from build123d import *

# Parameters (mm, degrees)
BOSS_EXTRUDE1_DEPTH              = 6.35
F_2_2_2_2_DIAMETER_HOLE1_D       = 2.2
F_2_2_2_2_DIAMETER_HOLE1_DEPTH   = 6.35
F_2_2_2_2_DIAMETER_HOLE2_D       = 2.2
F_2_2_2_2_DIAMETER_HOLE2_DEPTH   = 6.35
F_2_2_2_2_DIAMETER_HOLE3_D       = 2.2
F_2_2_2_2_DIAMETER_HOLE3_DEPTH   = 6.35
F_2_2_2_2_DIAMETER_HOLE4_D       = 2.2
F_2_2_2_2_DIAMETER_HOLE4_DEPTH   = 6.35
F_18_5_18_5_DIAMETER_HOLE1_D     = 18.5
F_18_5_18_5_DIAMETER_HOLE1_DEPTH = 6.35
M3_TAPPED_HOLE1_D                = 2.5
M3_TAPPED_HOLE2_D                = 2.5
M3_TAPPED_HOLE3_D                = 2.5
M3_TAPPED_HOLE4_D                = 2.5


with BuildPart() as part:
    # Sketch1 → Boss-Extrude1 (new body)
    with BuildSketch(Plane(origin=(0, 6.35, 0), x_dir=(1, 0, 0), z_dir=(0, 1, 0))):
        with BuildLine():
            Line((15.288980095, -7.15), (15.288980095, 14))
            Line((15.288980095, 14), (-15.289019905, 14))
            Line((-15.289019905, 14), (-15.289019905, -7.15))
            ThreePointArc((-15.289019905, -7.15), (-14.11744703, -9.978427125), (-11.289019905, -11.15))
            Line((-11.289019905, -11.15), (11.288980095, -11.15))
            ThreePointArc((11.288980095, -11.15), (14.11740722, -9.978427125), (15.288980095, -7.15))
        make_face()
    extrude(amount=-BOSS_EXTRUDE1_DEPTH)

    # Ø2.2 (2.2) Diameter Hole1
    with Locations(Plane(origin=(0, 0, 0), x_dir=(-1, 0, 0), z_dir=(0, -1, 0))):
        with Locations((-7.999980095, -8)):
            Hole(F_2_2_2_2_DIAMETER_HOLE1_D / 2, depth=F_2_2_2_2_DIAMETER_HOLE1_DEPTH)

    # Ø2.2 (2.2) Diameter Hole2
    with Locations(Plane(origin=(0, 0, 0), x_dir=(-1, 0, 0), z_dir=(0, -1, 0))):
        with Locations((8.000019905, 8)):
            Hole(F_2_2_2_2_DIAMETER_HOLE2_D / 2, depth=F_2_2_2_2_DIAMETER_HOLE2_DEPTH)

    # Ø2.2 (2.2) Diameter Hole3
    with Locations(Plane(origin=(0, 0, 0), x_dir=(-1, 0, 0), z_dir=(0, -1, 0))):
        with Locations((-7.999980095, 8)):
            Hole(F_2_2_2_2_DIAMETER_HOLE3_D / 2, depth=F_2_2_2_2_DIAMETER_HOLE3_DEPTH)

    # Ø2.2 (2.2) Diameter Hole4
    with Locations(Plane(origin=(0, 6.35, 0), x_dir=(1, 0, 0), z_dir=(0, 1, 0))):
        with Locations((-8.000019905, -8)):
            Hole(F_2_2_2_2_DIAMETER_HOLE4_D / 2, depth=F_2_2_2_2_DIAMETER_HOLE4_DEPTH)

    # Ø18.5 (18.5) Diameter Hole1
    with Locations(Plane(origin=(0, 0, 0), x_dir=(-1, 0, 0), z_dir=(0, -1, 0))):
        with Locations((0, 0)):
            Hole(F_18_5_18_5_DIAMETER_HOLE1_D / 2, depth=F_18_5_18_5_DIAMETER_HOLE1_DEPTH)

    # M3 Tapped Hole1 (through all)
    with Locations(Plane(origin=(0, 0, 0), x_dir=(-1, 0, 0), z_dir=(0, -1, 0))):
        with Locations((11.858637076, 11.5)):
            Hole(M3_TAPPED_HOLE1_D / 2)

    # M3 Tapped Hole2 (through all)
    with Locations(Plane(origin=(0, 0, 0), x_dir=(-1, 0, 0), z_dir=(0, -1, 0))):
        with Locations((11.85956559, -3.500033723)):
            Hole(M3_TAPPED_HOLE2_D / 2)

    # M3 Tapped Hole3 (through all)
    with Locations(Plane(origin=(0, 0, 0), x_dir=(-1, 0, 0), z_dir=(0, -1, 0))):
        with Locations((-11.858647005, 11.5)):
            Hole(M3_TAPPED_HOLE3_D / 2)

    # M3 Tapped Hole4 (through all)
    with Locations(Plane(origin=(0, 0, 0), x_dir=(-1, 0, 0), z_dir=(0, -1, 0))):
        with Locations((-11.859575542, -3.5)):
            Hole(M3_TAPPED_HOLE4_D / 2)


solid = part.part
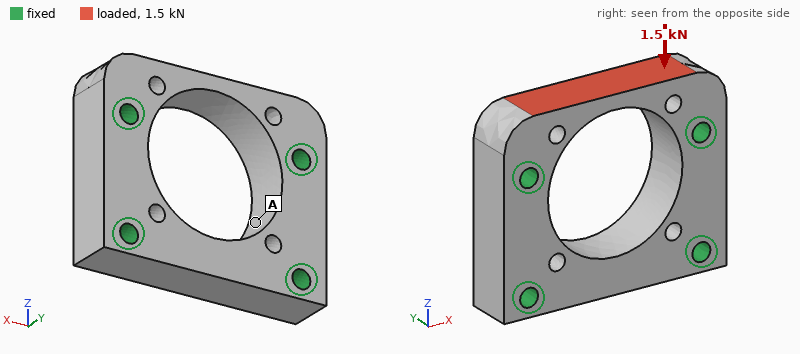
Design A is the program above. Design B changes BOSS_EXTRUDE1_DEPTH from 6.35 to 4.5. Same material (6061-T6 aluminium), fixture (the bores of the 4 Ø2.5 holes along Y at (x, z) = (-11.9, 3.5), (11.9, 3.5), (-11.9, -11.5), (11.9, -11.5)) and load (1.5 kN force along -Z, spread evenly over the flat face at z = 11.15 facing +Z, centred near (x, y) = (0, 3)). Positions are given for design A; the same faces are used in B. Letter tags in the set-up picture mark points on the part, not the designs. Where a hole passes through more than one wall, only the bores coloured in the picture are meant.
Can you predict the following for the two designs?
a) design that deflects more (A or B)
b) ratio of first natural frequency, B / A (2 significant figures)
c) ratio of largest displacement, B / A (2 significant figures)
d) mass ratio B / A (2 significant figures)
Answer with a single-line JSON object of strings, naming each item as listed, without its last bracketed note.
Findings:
{"design that deflects more": "B", "ratio of first natural frequency, B / A": "0.81", "ratio of largest displacement, B / A": "1.4", "mass ratio B / A": "0.71"}
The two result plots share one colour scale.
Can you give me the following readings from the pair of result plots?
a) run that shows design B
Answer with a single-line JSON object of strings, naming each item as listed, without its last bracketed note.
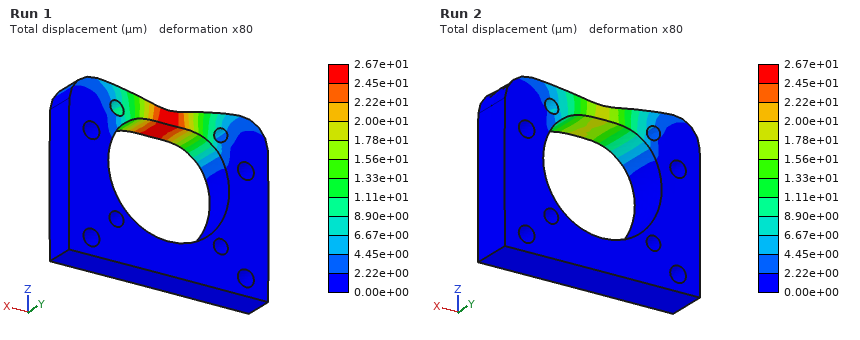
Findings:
{"run that shows design B": "Run 1"}
